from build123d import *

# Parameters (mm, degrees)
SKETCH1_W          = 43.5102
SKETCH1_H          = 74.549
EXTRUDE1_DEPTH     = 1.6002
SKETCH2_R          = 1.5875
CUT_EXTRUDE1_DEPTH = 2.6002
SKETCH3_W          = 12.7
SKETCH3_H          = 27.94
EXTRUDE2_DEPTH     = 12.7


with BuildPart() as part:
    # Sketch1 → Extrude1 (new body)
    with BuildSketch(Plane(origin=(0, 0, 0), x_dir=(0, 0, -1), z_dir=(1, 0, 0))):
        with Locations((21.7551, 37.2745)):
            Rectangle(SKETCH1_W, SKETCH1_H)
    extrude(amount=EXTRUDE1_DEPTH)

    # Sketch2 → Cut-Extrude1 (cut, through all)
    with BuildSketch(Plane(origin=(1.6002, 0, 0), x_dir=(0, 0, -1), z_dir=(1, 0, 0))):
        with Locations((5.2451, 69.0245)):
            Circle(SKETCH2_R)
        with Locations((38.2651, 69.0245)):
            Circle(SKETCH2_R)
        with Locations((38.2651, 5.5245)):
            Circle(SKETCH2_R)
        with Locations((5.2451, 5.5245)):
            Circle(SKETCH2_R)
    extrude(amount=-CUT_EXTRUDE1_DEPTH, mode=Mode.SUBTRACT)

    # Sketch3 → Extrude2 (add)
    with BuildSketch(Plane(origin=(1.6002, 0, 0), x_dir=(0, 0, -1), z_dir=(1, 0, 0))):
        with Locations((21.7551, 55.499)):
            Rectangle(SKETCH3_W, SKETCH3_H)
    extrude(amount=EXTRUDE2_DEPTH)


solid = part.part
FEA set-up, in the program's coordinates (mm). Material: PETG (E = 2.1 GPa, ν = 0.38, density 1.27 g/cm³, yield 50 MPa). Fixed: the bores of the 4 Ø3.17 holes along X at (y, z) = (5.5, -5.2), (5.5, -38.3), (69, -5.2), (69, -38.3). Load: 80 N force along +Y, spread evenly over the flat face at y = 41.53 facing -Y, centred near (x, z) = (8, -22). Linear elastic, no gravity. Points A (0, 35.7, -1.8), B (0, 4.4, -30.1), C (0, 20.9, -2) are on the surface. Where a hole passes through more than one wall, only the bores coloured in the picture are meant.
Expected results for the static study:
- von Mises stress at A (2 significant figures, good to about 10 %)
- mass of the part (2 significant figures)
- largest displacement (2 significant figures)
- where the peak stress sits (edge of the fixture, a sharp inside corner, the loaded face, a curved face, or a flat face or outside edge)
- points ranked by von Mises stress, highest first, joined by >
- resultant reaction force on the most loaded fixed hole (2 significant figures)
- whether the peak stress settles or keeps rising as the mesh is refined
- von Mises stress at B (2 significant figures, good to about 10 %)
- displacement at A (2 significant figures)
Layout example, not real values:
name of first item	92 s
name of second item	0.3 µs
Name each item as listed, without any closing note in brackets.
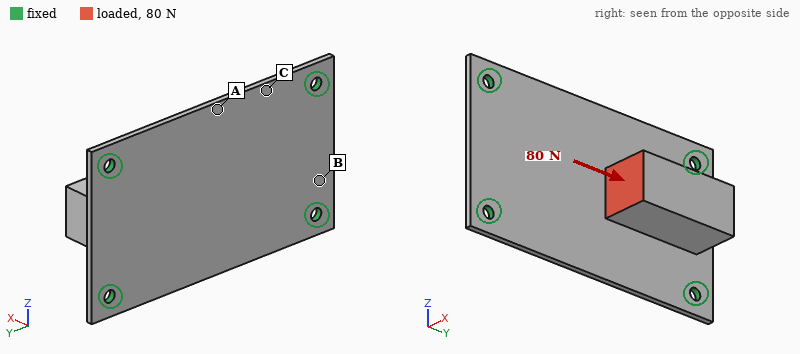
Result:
von Mises stress at A	5.6 MPa
mass of the part	12 g
largest displacement	0.91 mm
where the peak stress sits	edge of the fixture
points ranked by von Mises stress, highest first, joined by >	A > B > C
resultant reaction force on the most loaded fixed hole	27 N
whether the peak stress settles or keeps rising as the mesh is refined	keeps rising
von Mises stress at B	3.3 MPa
displacement at A	0.70 mm
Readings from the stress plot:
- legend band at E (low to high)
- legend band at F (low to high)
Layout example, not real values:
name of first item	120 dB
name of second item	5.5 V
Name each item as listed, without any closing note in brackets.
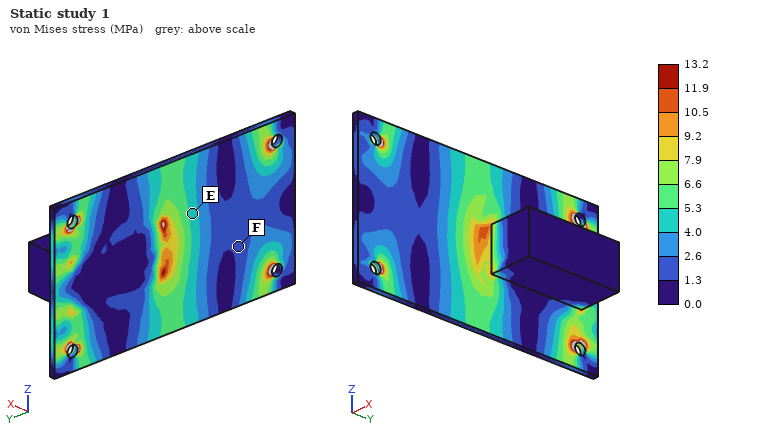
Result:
legend band at E	4.0 to 5.3 MPa
legend band at F	1.3 to 2.6 MPa
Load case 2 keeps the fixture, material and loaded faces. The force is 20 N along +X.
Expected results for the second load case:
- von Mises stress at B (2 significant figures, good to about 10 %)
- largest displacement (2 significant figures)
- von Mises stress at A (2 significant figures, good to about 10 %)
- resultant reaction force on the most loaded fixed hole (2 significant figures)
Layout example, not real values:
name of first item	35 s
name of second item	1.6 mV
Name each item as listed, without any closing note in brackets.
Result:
von Mises stress at B	2.9 MPa
largest displacement	0.85 mm
von Mises stress at A	5.2 MPa
resultant reaction force on the most loaded fixed hole	6.4 N
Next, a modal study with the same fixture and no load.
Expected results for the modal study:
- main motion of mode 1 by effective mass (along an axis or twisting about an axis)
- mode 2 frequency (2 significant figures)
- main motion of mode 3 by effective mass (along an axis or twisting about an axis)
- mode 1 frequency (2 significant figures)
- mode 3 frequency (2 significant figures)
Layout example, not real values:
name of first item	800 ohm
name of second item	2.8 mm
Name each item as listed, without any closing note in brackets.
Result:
main motion of mode 1 by effective mass	along X
mode 2 frequency	930 Hz
main motion of mode 3 by effective mass	along X
mode 1 frequency	380 Hz
mode 3 frequency	1200 Hz
